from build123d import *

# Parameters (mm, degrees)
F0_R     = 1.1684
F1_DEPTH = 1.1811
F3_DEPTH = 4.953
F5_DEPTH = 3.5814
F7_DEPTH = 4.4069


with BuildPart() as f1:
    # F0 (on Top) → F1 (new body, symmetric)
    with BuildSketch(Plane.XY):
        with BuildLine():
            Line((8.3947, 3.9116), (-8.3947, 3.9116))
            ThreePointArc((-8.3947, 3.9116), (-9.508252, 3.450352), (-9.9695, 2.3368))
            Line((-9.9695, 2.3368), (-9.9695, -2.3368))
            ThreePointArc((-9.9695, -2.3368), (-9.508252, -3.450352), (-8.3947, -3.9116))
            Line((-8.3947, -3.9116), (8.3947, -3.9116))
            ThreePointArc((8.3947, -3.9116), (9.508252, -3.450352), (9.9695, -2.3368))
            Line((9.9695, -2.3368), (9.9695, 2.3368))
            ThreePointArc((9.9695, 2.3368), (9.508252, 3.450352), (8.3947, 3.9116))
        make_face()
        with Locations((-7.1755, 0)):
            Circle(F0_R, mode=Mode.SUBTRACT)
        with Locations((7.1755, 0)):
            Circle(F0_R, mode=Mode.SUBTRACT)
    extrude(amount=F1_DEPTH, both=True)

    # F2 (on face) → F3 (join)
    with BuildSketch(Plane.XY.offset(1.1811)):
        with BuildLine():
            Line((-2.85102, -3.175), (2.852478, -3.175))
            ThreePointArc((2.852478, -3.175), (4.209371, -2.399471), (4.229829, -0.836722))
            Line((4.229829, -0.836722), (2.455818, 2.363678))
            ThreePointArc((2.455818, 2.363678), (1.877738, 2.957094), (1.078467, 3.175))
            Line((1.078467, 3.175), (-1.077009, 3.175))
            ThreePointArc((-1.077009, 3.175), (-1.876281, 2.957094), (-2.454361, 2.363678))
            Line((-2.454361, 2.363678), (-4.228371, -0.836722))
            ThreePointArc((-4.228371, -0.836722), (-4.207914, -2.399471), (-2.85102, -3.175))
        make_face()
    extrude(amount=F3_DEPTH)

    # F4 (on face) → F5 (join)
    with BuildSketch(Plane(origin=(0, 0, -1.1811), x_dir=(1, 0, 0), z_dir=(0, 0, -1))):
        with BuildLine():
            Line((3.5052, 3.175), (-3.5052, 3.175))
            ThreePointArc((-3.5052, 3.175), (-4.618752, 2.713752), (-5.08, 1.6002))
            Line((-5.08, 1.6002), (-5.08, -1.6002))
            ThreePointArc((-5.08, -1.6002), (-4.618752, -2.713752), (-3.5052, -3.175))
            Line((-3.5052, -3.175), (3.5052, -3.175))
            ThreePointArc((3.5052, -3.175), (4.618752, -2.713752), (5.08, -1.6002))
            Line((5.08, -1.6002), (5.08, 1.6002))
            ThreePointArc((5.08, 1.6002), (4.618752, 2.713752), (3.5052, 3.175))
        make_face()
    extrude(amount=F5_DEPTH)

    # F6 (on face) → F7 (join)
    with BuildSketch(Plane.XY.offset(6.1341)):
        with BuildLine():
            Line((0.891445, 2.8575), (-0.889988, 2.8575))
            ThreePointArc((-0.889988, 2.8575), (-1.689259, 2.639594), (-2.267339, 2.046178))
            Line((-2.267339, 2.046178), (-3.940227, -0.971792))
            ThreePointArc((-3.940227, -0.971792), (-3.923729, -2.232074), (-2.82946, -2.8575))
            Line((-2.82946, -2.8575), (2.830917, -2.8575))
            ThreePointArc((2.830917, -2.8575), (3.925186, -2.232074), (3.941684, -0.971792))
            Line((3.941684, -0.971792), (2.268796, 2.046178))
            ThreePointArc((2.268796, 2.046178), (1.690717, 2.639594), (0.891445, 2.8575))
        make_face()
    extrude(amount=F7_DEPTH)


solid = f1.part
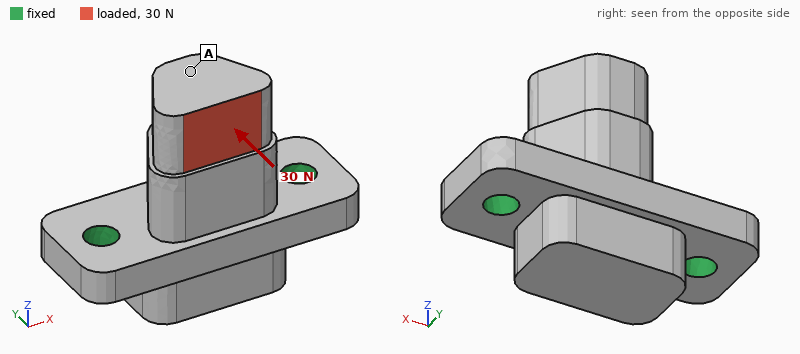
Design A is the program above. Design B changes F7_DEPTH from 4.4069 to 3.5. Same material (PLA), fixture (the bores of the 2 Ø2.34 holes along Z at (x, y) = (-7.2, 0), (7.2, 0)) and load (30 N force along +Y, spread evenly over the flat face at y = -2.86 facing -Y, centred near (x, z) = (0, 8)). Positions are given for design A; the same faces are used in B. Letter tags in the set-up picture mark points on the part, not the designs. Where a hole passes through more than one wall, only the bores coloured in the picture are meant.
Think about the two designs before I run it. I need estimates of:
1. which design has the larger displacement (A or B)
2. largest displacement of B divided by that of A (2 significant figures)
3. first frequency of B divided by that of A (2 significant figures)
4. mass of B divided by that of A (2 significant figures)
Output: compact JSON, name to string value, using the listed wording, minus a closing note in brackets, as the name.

{"which design has the larger displacement": "A", "largest displacement of B divided by that of A": "0.87", "first frequency of B divided by that of A": "1.1", "mass of B divided by that of A": "0.97"}
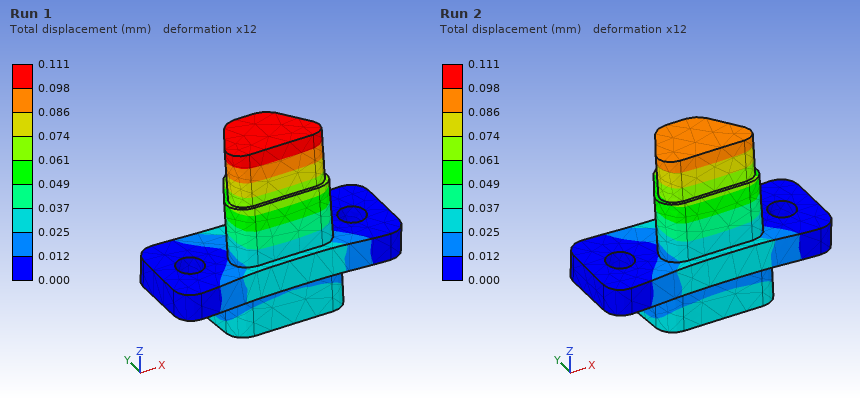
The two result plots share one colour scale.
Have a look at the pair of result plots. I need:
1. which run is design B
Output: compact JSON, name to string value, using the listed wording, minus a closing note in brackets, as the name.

{"which run is design B": "Run 2"}
